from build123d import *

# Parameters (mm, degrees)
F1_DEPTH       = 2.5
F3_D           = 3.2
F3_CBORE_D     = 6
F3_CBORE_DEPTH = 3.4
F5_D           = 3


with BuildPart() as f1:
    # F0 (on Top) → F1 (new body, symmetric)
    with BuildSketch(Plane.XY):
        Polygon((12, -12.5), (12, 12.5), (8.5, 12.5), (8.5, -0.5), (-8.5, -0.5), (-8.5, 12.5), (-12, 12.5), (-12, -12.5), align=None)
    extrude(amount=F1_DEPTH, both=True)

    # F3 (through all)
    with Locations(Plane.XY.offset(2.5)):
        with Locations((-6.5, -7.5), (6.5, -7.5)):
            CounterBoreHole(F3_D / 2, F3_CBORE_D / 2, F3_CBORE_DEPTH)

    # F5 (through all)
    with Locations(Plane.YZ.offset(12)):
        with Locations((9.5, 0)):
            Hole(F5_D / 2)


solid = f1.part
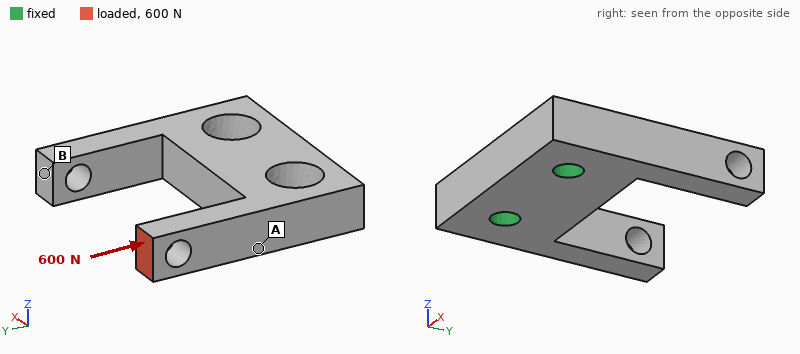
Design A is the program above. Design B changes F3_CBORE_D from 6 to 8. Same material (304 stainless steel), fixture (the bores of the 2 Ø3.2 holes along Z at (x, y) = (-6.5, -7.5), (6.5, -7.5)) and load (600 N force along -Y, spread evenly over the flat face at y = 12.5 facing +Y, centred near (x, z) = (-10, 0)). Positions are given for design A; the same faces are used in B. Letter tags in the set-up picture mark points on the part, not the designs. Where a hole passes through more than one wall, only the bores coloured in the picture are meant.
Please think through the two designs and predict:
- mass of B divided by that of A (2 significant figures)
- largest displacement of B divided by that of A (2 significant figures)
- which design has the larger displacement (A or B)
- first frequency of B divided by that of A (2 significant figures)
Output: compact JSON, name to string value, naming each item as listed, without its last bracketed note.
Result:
{"mass of B divided by that of A": "0.91", "largest displacement of B divided by that of A": "1.4", "which design has the larger displacement": "B", "first frequency of B divided by that of A": "0.90"}
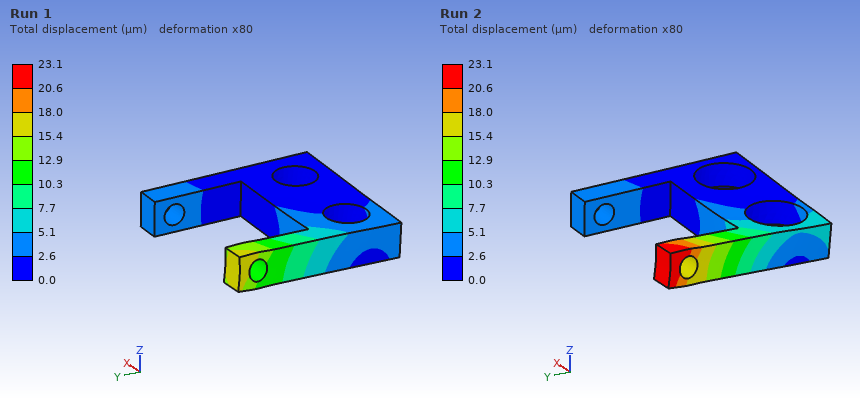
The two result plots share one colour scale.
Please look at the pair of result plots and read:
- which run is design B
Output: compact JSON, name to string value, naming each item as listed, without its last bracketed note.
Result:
{"which run is design B": "Run 2"}
